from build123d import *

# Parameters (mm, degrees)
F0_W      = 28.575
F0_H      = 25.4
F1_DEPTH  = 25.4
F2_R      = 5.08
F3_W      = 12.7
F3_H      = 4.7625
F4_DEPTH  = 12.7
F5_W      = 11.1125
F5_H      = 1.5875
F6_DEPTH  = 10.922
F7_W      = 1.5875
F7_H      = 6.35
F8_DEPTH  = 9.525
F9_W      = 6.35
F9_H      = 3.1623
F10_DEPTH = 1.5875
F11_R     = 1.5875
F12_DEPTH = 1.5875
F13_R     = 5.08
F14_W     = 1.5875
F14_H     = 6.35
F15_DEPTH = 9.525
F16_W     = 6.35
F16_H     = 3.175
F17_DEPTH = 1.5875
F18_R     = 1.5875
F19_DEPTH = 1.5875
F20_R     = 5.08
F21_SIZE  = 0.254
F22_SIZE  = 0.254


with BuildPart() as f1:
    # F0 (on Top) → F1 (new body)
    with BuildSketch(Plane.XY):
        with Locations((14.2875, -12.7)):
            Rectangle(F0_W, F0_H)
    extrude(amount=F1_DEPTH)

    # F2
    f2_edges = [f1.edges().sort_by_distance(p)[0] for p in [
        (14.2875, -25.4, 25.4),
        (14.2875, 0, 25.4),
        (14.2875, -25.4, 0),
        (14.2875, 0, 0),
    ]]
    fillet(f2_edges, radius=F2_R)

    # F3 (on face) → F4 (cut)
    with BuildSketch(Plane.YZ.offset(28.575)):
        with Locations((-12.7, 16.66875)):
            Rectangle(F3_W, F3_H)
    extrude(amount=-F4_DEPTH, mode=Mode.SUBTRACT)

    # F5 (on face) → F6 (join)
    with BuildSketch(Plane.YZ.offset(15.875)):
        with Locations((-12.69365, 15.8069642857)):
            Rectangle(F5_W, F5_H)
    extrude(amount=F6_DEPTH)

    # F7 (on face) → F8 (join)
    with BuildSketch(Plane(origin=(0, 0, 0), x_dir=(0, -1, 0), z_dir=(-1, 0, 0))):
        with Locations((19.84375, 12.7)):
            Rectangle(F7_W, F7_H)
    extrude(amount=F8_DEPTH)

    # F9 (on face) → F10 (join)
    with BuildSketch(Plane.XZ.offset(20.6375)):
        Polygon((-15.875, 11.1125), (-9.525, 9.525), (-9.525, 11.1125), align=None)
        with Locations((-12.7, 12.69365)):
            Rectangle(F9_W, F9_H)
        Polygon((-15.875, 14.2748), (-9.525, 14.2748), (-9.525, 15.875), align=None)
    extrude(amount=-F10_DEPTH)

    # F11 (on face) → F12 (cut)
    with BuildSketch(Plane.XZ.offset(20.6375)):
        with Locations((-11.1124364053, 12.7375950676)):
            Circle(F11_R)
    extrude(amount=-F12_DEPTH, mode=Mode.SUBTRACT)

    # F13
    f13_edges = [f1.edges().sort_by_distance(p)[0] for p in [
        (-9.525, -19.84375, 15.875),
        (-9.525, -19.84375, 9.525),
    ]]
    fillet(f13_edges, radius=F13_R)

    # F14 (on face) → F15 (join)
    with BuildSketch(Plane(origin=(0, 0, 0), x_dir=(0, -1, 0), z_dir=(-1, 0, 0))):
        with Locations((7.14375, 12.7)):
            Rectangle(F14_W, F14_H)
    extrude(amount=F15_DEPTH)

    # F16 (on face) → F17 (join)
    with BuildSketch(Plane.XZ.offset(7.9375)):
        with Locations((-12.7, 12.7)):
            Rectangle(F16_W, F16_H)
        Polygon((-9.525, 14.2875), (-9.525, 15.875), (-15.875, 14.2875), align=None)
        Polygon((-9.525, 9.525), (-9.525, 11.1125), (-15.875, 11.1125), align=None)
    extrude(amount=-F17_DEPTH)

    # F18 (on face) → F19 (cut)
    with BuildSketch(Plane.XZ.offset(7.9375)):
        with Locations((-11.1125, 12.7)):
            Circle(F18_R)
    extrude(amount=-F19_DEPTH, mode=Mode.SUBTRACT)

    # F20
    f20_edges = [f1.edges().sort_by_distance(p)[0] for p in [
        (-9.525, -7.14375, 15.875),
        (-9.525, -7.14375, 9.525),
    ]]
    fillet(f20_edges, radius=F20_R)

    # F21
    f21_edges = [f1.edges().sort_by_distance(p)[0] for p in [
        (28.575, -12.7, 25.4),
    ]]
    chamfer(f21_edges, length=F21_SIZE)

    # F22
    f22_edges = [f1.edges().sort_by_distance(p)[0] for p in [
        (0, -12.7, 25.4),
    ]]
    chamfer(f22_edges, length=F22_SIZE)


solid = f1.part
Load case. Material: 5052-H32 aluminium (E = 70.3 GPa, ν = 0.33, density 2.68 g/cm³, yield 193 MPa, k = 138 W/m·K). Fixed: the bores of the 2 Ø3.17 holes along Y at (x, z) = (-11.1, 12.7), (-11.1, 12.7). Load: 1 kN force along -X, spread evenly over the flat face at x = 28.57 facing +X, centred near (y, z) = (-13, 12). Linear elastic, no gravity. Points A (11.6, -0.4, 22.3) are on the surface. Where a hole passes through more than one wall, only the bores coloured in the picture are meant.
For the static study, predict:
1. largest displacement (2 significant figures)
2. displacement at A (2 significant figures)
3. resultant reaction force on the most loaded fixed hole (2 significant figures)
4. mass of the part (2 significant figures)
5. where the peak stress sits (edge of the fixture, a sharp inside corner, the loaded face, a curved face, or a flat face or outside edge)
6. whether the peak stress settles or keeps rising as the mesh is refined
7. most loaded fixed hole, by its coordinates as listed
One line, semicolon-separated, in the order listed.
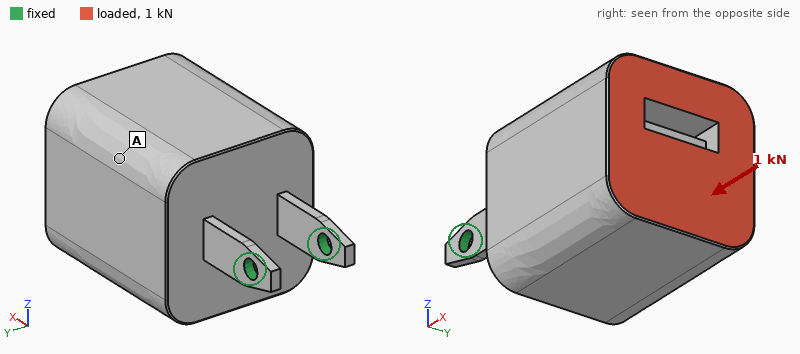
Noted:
49 µm; 21 µm; 560 N; 47 g; edge of the fixture; keeps rising; (-11.1, 12.7)
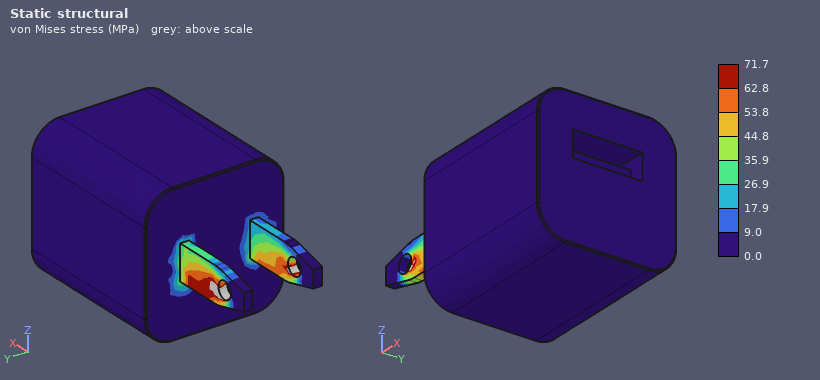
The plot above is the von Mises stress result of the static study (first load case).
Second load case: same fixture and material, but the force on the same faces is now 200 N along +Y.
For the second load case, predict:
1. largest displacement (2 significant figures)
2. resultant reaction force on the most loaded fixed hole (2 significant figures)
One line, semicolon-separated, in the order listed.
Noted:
0.11 mm; 530 N
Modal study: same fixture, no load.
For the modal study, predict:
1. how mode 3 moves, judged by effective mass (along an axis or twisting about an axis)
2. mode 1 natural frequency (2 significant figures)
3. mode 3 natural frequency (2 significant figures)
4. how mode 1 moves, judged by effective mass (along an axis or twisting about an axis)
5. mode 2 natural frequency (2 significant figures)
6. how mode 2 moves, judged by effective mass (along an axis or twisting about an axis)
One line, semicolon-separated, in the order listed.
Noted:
twisting about X; 630 Hz; 2000 Hz; along Z; 1200 Hz; along Y
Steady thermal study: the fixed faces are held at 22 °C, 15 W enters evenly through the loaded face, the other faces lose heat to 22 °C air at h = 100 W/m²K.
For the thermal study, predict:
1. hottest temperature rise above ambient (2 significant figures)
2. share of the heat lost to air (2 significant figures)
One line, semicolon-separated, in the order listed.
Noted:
26 K; 64 %
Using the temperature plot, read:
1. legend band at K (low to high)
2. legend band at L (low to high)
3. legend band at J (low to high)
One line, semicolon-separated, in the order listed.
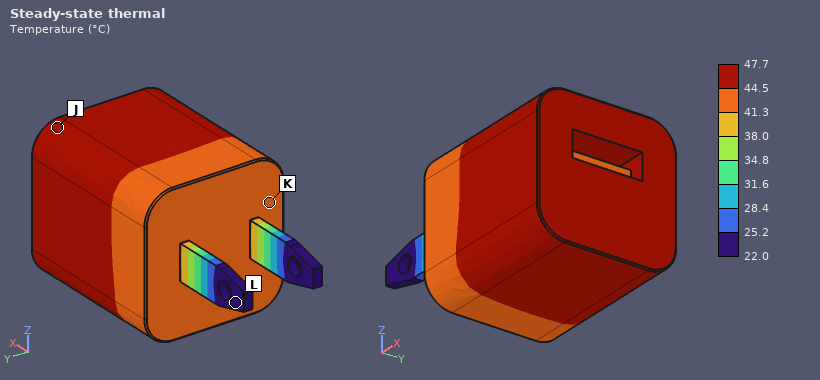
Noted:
41.3 to 44.5 °C; 22.0 to 25.2 °C; 44.5 to 47.7 °C
